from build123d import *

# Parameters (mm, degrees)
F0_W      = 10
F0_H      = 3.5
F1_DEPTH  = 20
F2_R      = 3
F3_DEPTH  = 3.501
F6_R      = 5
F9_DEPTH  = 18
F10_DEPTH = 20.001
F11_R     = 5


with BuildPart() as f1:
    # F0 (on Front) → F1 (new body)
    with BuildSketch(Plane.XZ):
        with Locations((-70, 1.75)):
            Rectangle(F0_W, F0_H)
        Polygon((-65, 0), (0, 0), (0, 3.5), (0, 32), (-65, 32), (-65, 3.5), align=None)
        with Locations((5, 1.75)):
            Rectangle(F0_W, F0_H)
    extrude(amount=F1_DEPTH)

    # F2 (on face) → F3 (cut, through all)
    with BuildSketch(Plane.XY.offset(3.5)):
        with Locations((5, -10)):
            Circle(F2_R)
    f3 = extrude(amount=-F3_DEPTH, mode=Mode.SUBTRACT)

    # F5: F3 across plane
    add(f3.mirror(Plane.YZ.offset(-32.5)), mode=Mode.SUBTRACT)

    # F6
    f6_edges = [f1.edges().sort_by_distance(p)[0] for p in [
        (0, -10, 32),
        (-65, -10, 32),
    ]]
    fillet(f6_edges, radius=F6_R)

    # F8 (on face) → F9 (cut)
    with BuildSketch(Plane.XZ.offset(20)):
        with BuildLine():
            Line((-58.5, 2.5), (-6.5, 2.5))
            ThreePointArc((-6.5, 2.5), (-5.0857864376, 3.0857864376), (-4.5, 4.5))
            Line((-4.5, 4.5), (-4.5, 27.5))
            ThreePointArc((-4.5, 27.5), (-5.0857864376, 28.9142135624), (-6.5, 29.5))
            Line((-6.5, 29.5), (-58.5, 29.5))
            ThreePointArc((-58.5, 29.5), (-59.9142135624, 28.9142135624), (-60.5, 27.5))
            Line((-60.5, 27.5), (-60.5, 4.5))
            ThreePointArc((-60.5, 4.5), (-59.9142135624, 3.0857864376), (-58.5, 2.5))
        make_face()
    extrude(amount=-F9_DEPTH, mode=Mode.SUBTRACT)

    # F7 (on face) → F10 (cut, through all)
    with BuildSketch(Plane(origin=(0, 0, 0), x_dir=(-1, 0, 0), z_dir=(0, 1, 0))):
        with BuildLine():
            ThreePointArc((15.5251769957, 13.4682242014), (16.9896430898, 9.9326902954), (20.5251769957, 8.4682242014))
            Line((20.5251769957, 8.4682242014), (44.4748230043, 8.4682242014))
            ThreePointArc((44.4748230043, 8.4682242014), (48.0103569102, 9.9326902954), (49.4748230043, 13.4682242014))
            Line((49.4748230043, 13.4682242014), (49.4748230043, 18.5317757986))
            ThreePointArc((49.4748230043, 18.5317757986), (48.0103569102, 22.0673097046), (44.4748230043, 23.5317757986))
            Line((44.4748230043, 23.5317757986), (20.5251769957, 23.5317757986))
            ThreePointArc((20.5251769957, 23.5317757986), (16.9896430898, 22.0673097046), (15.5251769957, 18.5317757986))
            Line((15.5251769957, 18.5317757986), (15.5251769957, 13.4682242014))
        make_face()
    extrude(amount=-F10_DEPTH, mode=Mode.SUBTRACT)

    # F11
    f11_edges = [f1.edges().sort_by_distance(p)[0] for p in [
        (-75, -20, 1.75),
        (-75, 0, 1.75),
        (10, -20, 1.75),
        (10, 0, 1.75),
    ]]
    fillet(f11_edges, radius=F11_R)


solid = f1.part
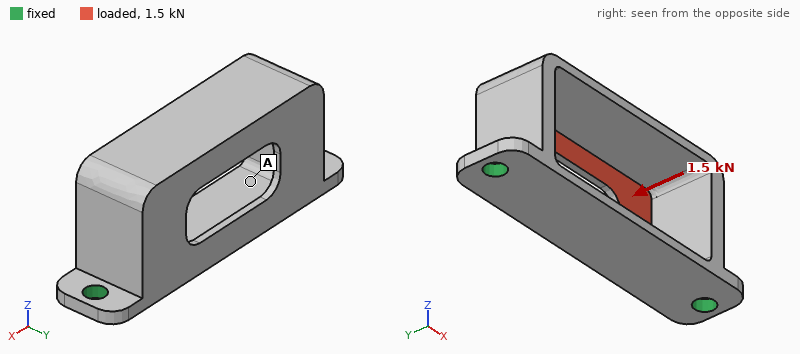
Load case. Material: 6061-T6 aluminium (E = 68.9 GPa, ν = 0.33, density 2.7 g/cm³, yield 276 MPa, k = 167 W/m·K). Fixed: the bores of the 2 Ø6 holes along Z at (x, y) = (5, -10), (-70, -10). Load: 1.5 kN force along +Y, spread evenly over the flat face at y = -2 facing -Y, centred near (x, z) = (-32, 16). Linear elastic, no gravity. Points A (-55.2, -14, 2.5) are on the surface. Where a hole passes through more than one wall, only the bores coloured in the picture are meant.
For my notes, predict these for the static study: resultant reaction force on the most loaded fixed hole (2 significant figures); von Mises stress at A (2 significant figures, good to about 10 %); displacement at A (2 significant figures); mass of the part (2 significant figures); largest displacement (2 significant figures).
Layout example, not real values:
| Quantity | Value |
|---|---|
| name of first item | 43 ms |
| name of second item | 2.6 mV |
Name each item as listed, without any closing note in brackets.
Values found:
| Quantity | Value |
|---|---|
| resultant reaction force on the most loaded fixed hole | 750 N |
| von Mises stress at A | 22 MPa |
| displacement at A | 0.032 mm |
| mass of the part | 39 g |
| largest displacement | 0.17 mm |
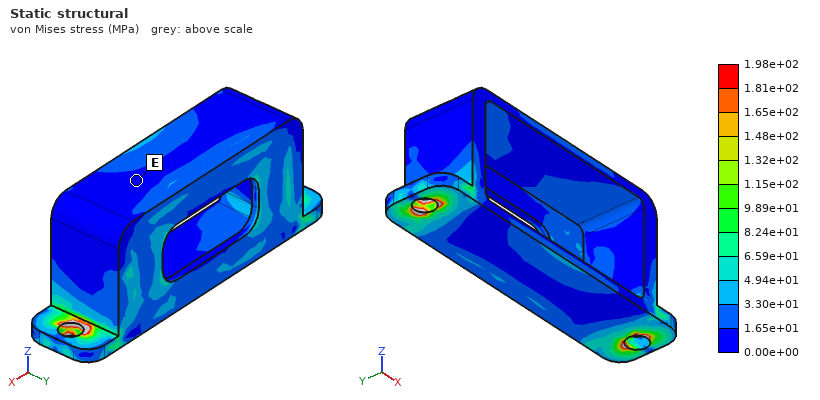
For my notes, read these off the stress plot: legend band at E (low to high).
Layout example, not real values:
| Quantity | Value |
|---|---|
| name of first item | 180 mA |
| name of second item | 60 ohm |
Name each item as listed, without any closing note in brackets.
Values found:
| Quantity | Value |
|---|---|
| legend band at E | 0.00e+00 to 1.65e+01 MPa |
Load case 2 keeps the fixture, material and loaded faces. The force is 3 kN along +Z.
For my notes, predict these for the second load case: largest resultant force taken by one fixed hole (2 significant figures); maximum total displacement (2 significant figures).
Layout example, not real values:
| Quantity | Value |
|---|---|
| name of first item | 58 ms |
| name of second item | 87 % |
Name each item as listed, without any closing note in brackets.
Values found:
| Quantity | Value |
|---|---|
| largest resultant force taken by one fixed hole | 1.6 kN |
| maximum total displacement | 0.19 mm |
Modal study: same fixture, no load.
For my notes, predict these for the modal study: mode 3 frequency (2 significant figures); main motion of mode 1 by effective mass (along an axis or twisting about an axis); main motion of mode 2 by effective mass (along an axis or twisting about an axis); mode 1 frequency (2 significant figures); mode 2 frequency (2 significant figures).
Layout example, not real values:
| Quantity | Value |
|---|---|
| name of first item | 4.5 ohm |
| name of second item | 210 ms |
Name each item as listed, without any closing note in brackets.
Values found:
| Quantity | Value |
|---|---|
| mode 3 frequency | 5400 Hz |
| main motion of mode 1 by effective mass | along Y |
| main motion of mode 2 by effective mass | along X |
| mode 1 frequency | 2800 Hz |
| mode 2 frequency | 3600 Hz |
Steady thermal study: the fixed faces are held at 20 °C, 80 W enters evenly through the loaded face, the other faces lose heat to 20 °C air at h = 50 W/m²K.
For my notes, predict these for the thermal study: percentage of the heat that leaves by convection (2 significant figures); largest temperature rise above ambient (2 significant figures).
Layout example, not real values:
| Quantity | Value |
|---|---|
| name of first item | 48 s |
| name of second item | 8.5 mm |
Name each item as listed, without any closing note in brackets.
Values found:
| Quantity | Value |
|---|---|
| percentage of the heat that leaves by convection | 21 % |
| largest temperature rise above ambient | 60 K |
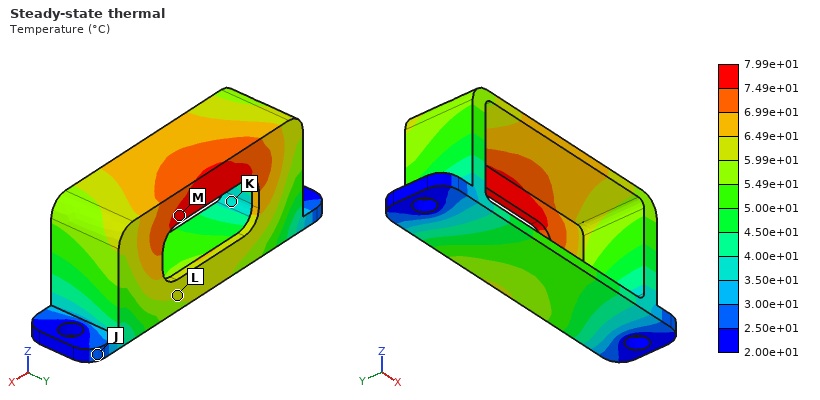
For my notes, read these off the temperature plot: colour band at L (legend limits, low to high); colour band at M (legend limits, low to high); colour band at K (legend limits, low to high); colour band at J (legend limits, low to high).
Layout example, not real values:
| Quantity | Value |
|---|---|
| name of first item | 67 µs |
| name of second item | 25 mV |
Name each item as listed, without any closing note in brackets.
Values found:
| Quantity | Value |
|---|---|
| colour band at L | 5.99e+01 to 6.49e+01 °C |
| colour band at M | 7.49e+01 to 7.99e+01 °C |
| colour band at K | 3.50e+01 to 4.00e+01 °C |
| colour band at J | 2.50e+01 to 3.00e+01 °C |
